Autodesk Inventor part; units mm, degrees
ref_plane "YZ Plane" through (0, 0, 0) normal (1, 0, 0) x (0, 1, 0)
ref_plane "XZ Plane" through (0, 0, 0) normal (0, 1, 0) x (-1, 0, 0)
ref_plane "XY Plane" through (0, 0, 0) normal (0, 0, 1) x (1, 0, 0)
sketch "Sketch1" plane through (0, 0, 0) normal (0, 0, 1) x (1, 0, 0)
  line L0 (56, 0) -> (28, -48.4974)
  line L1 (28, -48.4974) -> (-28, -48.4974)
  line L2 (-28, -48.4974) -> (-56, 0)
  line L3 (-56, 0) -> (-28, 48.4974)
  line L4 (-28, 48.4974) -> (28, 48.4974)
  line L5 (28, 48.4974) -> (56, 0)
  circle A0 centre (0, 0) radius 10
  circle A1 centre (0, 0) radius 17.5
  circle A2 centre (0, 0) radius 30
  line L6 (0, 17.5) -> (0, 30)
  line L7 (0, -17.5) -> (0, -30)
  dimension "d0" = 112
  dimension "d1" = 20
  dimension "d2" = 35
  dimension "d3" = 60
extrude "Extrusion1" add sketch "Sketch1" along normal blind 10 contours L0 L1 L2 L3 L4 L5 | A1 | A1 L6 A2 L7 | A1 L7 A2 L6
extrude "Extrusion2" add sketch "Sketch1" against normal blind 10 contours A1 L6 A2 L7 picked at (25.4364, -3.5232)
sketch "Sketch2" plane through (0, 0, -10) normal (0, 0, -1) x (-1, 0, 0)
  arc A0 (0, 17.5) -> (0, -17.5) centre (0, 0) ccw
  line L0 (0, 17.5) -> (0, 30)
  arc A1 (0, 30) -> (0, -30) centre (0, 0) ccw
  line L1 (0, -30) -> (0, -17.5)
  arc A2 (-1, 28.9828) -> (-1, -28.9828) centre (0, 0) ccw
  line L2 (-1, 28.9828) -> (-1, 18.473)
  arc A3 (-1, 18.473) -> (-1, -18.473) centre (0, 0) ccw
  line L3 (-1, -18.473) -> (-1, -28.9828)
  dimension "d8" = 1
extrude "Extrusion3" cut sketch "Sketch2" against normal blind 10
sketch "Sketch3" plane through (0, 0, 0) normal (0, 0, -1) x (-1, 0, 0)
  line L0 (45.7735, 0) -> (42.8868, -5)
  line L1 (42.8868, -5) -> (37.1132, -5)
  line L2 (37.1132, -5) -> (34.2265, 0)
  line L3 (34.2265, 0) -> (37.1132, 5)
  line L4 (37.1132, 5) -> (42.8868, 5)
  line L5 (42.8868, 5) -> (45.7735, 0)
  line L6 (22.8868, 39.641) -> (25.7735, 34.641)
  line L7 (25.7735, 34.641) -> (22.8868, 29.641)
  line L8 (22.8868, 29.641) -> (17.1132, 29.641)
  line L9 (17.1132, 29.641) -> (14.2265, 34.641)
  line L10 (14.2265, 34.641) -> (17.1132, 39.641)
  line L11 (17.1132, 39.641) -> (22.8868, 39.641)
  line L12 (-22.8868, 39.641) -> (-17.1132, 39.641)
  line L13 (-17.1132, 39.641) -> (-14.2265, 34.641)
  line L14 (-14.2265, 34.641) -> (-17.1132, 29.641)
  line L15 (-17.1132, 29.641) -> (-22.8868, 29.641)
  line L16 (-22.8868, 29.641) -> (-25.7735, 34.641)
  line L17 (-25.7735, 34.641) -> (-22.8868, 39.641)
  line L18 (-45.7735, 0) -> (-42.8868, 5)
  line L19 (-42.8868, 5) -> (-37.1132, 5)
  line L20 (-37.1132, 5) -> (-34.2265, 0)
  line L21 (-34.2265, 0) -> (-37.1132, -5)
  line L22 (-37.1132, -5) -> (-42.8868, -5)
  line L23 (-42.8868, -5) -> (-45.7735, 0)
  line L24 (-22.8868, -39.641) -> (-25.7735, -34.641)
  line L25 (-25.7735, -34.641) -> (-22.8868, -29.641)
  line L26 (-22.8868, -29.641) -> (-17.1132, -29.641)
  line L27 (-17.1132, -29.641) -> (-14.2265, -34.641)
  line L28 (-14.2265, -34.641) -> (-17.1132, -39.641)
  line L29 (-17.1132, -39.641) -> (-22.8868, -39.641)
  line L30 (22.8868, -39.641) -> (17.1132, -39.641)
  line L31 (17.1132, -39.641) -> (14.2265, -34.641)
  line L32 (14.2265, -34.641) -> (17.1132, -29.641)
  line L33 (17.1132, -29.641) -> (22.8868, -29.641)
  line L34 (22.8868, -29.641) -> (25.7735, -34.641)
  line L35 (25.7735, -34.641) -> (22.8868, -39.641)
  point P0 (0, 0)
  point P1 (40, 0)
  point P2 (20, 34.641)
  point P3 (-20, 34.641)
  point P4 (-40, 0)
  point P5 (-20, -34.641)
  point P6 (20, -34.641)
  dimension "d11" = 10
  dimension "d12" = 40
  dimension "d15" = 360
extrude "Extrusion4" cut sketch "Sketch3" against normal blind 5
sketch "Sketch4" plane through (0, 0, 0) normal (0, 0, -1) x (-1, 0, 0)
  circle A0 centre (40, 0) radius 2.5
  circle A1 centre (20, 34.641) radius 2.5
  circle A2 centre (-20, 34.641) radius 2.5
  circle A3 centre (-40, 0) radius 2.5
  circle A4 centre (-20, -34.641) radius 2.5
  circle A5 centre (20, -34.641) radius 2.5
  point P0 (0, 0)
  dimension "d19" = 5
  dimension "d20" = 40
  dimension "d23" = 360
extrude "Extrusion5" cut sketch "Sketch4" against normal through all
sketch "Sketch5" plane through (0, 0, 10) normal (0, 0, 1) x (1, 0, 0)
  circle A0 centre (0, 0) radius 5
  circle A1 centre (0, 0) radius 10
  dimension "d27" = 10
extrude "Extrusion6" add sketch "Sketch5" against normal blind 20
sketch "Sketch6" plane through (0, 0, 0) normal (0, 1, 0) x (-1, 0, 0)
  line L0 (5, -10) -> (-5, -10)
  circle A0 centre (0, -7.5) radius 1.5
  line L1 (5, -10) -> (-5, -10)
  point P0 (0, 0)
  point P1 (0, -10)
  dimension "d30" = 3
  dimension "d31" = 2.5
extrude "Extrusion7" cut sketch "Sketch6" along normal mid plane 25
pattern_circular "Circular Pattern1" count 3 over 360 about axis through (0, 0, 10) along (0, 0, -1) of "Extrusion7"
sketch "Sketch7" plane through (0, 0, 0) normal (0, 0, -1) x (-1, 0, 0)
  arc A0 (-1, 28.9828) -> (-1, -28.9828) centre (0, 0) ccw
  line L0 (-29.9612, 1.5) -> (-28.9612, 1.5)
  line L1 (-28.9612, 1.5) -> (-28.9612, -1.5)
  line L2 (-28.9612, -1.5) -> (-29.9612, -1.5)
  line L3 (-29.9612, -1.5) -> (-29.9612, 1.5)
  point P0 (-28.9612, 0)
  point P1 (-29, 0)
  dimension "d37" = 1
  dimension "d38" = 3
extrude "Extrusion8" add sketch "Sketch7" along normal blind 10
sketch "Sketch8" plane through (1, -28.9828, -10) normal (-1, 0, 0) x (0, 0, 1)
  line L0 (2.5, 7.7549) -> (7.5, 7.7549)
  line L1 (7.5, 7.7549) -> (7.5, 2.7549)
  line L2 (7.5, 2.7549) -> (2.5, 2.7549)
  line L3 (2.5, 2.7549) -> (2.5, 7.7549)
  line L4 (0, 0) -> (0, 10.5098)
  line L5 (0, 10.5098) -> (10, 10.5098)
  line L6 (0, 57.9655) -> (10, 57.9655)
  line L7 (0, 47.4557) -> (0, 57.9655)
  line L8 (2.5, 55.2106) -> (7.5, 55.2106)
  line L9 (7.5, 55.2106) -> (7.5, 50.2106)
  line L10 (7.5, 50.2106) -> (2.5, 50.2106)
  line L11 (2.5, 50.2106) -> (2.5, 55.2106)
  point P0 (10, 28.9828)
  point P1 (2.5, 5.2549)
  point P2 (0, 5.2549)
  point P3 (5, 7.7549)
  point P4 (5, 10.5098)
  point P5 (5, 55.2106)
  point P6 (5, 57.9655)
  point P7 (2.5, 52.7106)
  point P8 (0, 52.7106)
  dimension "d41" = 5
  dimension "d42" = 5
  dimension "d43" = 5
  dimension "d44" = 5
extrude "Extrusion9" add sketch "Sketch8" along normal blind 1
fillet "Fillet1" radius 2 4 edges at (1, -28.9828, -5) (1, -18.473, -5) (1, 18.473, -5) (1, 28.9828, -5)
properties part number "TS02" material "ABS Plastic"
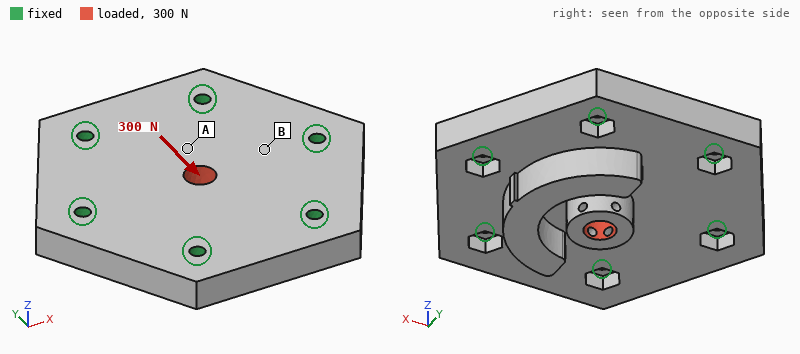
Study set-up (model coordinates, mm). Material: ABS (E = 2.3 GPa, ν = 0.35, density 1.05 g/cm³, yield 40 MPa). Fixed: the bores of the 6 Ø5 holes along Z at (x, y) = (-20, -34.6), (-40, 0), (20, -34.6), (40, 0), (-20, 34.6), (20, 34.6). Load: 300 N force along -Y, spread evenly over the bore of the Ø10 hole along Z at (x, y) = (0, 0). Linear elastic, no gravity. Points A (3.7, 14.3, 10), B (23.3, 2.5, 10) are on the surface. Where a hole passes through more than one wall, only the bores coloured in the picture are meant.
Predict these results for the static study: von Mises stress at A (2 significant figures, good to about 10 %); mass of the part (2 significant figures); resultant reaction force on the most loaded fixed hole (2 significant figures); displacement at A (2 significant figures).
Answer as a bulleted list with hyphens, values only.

- 0.40 MPa
- 92 g
- 69 N
- 7.1 µm
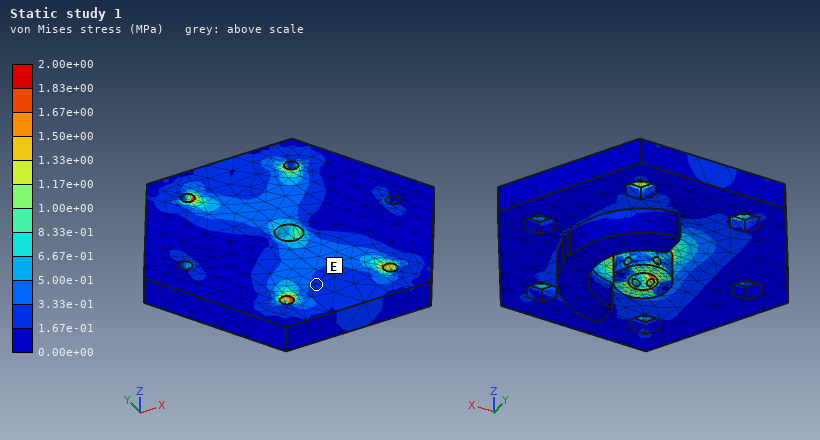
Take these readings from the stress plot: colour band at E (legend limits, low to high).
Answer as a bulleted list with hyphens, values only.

- 1.67e-01 to 3.33e-01 MPa
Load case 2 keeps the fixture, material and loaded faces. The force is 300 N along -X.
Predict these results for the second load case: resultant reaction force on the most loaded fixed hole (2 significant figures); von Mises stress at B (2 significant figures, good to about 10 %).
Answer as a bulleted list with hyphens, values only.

- 79 N
- 0.49 MPa
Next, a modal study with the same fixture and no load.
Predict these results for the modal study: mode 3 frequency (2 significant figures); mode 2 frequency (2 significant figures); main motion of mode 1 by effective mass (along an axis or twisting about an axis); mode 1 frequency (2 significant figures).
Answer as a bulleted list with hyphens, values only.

- 4600 Hz
- 4500 Hz
- along Z
- 2700 Hz
